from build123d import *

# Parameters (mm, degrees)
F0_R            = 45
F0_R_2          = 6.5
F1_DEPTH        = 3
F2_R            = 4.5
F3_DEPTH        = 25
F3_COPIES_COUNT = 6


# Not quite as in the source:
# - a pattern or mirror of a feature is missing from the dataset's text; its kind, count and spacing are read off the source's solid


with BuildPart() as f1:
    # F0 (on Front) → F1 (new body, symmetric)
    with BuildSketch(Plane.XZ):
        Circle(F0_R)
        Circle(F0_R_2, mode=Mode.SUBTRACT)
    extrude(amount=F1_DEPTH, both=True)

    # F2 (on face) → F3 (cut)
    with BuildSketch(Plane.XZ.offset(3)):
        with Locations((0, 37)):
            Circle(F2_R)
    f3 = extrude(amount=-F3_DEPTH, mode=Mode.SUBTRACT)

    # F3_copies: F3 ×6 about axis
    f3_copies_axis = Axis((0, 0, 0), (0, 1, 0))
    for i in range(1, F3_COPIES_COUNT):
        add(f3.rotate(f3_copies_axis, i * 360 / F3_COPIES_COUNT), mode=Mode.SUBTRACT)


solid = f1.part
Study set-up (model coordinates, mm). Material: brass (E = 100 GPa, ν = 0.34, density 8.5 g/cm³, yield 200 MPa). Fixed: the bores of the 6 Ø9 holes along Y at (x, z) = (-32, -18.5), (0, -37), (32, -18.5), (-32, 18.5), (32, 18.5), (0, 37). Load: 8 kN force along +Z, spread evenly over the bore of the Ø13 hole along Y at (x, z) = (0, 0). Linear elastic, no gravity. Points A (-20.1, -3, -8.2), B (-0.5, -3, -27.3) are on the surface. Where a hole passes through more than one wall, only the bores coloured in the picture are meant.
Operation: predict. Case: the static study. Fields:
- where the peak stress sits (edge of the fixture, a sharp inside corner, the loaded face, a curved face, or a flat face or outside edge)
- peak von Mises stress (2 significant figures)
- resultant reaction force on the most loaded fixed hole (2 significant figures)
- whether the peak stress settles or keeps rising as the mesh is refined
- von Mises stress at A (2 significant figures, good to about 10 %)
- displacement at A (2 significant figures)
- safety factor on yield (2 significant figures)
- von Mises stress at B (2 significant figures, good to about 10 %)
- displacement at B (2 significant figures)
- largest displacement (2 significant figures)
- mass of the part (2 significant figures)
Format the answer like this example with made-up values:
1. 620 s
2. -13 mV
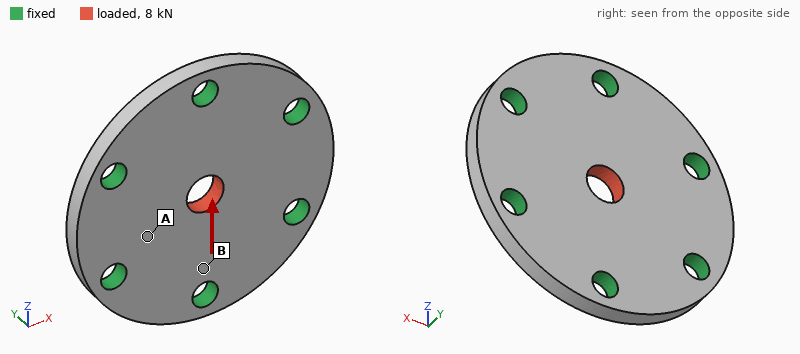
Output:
1. the loaded face
2. 57 MPa
3. 2.2 kN
4. settles
5. 10 MPa
6. 1.5 µm
7. 3.5
8. 24 MPa
9. 1.3 µm
10. 6.5 µm
11. 300 g
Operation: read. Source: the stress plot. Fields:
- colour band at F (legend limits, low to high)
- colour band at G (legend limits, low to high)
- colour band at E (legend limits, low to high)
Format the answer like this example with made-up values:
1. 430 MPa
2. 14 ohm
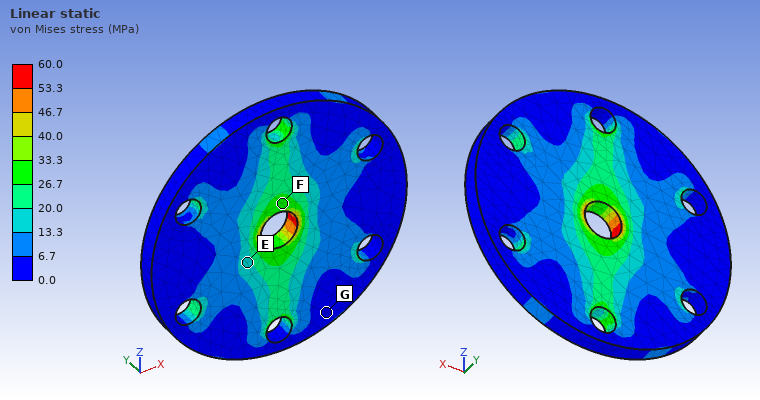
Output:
1. 26.7 to 33.3 MPa
2. 0.0 to 6.7 MPa
3. 13.3 to 20.0 MPa
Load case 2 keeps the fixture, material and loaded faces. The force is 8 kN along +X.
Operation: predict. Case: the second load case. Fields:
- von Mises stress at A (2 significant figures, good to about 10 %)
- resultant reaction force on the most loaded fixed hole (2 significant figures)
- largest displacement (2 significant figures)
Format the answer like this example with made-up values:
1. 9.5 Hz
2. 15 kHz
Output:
1. 18 MPa
2. 1.9 kN
3. 6.5 µm
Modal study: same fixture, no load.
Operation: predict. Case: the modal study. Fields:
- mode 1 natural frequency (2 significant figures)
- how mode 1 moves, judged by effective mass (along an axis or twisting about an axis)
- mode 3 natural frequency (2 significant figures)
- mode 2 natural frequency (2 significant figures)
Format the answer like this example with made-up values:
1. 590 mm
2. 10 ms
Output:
1. 7200 Hz
2. along Y
3. 13 kHz
4. 13 kHz
